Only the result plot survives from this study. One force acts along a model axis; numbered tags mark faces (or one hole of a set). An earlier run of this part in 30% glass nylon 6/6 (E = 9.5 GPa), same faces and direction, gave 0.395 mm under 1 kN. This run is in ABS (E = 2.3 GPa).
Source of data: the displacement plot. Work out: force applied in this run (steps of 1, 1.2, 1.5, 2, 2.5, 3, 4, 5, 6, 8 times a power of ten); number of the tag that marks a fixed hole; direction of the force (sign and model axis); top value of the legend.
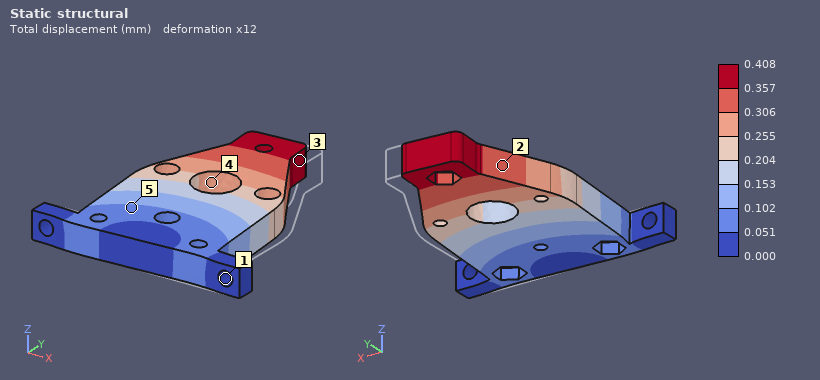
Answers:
250 N
1
-X
0.408 mm
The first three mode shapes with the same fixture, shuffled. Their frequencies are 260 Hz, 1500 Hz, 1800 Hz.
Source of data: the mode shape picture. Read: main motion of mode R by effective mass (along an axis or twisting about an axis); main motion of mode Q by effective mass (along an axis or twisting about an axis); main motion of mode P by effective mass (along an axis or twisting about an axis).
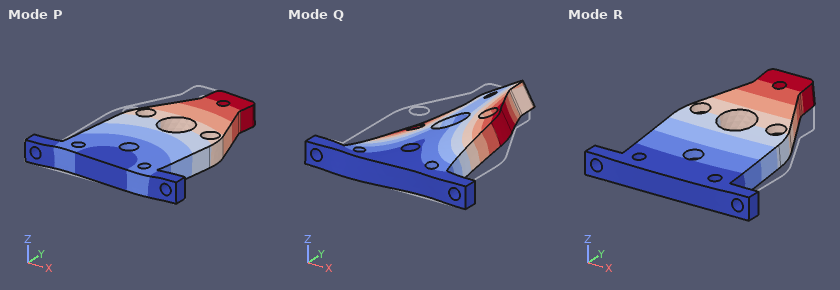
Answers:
along Z
twisting about Y
along X
